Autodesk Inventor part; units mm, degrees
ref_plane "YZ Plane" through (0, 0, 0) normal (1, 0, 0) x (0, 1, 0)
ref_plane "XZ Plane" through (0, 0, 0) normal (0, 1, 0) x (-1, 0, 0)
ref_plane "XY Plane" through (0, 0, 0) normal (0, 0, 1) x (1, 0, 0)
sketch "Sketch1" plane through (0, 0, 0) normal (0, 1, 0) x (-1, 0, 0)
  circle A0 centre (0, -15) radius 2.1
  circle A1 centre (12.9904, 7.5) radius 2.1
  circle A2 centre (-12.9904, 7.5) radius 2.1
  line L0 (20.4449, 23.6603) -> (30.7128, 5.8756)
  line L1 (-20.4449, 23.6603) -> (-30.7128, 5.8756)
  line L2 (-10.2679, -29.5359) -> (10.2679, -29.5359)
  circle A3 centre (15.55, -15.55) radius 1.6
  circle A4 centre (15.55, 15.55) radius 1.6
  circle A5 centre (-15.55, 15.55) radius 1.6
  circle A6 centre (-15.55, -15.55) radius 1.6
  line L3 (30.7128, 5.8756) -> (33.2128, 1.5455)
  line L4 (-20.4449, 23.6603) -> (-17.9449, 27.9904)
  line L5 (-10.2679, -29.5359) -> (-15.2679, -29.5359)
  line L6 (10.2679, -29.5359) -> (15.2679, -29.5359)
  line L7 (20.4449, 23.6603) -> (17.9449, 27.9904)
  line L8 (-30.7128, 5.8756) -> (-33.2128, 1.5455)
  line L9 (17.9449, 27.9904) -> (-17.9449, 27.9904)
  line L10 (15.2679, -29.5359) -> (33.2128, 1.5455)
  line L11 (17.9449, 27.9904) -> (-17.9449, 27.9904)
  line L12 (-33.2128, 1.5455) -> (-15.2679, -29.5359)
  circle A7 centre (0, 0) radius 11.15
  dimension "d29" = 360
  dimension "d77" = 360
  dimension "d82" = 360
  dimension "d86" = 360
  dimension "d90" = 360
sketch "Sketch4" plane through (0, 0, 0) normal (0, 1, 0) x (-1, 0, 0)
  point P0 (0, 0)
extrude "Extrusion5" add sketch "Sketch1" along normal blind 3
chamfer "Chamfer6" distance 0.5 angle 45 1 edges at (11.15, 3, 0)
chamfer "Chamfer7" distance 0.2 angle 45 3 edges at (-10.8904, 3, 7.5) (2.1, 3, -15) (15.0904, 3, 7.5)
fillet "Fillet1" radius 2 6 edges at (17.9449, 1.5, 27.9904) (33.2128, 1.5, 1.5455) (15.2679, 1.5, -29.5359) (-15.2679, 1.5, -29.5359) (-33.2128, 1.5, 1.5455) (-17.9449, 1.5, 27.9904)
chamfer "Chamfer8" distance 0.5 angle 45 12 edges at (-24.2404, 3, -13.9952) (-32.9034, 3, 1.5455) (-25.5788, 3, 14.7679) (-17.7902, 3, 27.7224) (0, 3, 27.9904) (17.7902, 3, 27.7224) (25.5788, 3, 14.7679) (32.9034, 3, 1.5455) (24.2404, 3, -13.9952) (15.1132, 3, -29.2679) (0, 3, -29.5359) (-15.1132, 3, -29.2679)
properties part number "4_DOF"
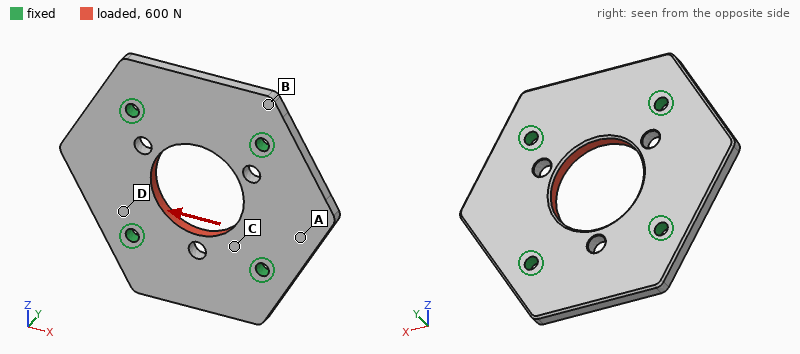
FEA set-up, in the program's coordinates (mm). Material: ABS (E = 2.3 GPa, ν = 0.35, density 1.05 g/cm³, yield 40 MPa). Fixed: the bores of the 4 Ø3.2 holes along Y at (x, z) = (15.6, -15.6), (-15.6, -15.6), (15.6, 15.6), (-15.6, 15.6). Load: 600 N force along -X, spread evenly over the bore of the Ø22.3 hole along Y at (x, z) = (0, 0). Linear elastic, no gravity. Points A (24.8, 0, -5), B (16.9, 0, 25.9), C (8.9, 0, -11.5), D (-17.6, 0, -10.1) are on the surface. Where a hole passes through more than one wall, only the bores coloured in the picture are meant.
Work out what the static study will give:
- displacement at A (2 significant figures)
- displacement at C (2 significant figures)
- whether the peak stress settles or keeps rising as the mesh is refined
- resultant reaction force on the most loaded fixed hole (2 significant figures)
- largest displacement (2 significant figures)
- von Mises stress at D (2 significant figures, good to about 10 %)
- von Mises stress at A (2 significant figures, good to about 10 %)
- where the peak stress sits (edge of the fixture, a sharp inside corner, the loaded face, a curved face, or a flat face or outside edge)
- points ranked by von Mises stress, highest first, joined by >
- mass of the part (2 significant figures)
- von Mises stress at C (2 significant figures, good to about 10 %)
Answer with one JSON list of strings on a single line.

["27 µm", "18 µm", "keeps rising", "150 N", "44 µm", "3.3 MPa", "1.8 MPa", "edge of the fixture", "C > D > A > B", "7.5 g", "4.3 MPa"]
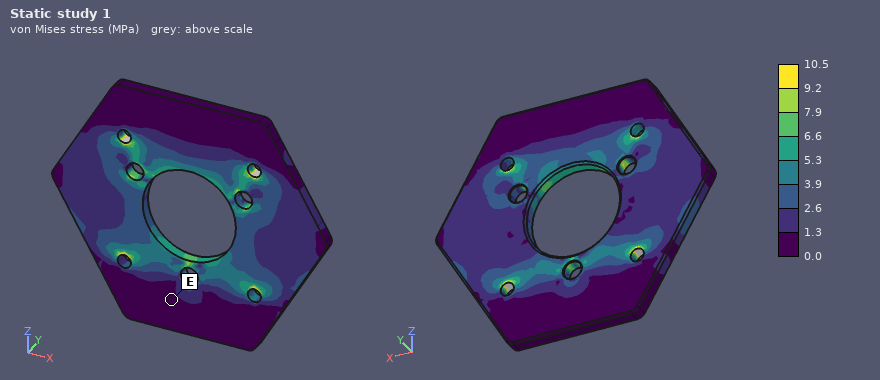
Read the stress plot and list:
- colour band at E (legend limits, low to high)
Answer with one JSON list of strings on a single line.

["0.0 to 1.3 MPa"]
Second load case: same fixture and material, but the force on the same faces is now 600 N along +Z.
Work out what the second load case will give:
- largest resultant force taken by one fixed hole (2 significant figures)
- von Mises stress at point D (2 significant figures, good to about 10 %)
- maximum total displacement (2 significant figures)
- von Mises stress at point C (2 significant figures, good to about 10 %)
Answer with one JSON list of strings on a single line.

["160 N", "2.5 MPa", "51 µm", "3.4 MPa"]
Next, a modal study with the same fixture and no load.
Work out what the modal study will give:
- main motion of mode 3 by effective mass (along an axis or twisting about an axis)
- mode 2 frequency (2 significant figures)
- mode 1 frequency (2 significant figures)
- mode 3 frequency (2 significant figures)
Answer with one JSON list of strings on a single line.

["along Y", "2600 Hz", "2600 Hz", "2900 Hz"]
